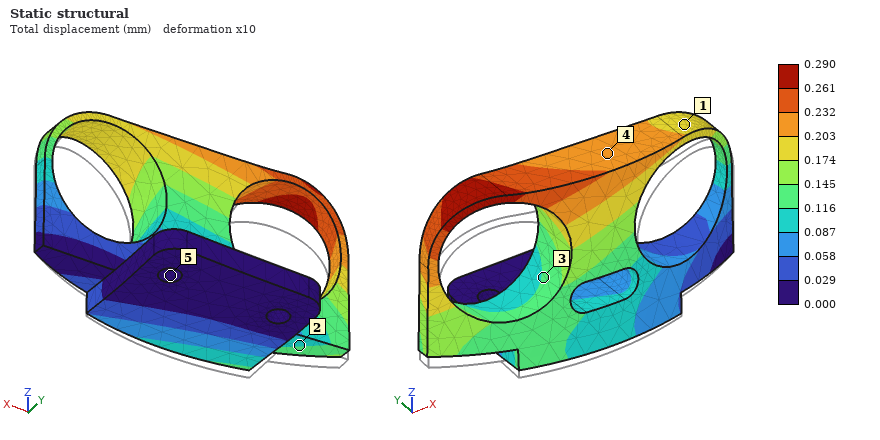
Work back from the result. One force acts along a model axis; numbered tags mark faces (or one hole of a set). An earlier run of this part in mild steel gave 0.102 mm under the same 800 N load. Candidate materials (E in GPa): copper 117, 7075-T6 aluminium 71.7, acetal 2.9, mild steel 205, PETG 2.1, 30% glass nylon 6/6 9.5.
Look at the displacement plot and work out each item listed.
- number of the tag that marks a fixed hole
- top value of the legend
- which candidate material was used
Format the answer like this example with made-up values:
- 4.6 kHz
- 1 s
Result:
- 5
- 0.290 mm
- 7075-T6 aluminium
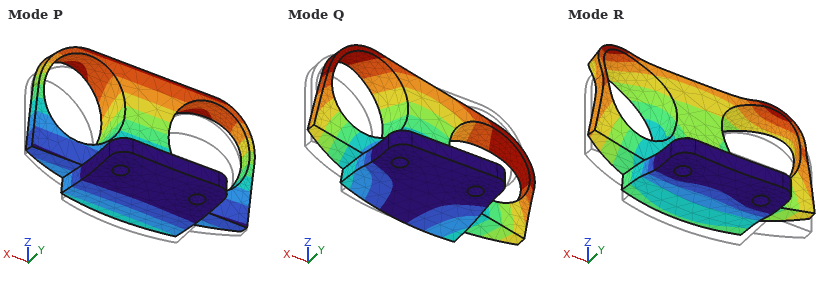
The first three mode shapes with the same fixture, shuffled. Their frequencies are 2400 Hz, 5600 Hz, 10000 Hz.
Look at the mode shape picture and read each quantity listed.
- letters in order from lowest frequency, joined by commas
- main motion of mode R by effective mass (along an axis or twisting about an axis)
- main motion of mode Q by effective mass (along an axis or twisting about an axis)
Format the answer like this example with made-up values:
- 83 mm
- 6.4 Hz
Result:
- P, Q, R
- along Z
- along X
